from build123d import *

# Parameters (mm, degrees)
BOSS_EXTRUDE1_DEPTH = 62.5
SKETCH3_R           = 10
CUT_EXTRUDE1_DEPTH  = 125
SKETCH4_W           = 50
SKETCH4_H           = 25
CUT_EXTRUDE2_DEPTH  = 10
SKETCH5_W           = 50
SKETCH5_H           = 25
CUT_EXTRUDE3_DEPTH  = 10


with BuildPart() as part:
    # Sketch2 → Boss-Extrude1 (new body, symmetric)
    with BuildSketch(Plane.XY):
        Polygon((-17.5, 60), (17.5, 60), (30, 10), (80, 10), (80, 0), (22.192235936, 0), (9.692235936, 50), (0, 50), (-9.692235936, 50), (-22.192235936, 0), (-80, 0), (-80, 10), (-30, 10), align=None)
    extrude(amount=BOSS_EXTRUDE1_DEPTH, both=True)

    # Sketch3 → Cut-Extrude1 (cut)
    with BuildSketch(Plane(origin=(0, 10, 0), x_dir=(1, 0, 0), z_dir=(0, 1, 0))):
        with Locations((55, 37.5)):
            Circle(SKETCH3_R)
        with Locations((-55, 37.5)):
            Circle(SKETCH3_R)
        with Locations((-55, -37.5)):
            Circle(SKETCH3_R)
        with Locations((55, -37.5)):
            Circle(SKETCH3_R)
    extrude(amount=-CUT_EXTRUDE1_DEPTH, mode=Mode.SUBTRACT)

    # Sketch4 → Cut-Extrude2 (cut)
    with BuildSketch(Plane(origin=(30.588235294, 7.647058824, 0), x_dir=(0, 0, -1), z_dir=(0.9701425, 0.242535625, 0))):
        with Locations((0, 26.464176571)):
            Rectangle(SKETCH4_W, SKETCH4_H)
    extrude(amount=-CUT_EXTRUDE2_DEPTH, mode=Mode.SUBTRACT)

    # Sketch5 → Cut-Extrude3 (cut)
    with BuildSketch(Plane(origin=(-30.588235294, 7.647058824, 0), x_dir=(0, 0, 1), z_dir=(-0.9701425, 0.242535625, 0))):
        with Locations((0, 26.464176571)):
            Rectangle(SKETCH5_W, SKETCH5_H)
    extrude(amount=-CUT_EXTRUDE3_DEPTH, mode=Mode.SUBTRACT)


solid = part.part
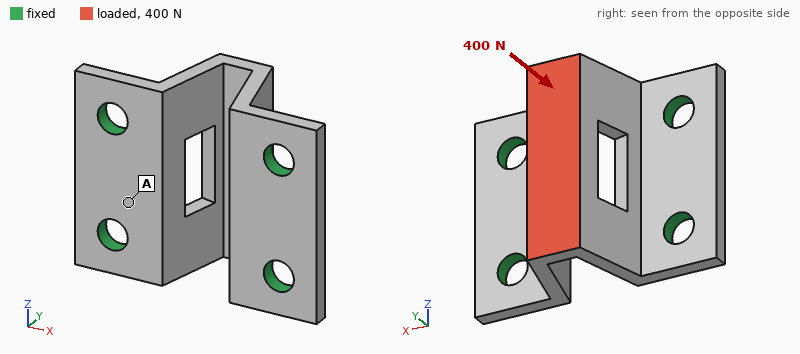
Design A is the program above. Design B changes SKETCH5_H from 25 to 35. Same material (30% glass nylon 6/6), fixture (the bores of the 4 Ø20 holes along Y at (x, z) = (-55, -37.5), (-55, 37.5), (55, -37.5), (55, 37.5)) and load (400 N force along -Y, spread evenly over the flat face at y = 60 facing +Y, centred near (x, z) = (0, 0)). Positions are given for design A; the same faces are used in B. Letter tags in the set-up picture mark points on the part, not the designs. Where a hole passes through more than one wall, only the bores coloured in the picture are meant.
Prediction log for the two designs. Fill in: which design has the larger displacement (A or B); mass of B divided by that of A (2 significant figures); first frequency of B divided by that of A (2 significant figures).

B
0.98
0.97
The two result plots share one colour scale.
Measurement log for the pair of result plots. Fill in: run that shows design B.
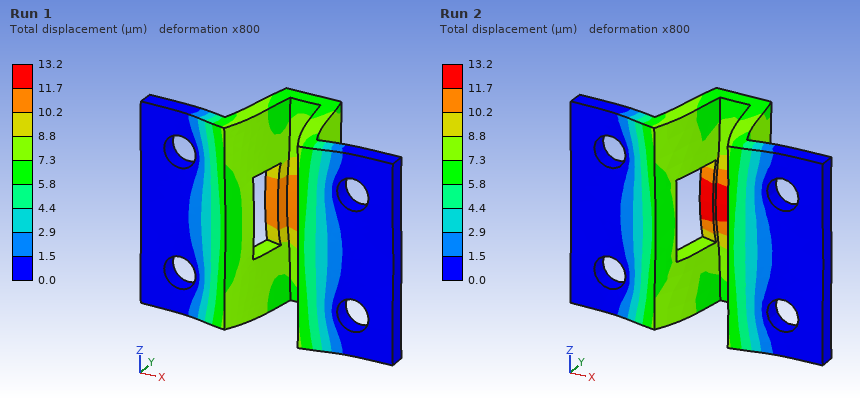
Run 2
